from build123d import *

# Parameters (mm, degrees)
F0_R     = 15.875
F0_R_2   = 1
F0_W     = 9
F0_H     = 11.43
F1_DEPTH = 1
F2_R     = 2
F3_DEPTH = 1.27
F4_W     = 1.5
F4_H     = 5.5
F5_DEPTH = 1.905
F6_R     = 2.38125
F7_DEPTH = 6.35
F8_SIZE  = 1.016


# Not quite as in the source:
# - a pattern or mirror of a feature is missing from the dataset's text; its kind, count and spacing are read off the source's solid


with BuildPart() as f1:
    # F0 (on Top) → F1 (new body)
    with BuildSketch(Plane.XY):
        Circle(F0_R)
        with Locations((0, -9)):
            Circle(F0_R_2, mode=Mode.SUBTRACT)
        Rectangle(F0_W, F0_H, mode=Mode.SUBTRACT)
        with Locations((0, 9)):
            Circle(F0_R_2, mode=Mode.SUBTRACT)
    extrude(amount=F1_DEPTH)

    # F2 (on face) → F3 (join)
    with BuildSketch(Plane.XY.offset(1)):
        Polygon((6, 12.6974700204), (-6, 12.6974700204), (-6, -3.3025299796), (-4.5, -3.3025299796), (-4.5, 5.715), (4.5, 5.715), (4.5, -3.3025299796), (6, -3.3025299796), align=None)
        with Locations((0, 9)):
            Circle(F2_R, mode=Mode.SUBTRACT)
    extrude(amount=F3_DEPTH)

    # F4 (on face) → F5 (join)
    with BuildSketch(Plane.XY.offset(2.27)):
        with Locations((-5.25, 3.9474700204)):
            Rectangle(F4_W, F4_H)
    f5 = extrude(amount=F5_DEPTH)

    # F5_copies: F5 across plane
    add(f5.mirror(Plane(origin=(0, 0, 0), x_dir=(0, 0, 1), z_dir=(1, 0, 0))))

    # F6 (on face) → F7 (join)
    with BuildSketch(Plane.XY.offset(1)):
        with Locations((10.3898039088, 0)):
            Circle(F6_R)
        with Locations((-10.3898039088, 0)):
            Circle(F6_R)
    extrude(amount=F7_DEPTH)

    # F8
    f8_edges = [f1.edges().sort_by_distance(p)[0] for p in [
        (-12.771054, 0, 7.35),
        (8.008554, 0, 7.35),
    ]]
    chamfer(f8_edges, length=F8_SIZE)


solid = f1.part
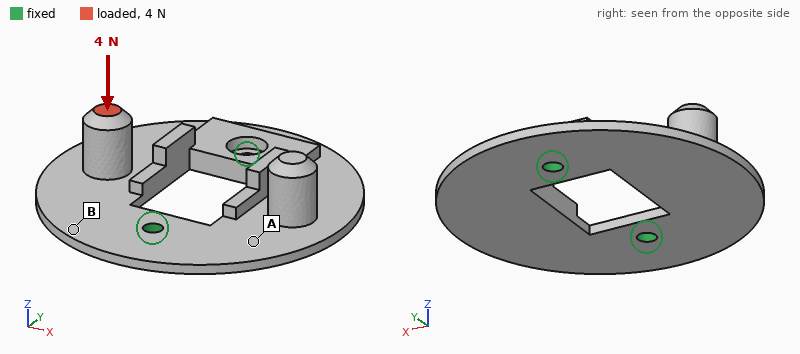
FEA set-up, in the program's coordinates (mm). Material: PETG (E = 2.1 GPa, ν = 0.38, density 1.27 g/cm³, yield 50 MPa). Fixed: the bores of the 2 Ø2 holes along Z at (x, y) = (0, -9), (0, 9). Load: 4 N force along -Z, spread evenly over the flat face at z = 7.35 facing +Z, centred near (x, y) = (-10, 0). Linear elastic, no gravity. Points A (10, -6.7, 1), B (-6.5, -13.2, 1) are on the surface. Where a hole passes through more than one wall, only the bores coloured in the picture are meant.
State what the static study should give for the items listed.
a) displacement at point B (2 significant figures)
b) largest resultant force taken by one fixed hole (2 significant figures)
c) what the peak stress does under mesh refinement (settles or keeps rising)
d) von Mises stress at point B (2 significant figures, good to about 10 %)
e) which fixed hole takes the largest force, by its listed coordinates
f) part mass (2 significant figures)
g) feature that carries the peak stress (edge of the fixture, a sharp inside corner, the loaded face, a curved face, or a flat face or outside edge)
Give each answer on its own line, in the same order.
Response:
0.087 mm
2.4 N
keeps rising
3.5 MPa
(0, 9)
1.3 g
edge of the fixture
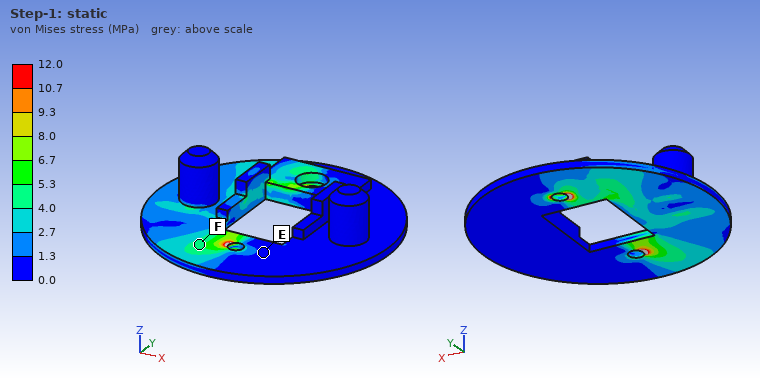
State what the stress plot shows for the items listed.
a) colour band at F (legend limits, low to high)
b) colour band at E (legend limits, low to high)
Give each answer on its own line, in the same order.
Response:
4.0 to 5.3 MPa
0.0 to 1.3 MPa
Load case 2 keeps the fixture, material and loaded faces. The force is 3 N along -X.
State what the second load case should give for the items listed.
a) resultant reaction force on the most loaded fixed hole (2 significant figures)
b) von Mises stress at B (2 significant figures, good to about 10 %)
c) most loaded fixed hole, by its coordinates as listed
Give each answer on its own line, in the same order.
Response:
1.8 N
2.8 MPa
(0, 9)
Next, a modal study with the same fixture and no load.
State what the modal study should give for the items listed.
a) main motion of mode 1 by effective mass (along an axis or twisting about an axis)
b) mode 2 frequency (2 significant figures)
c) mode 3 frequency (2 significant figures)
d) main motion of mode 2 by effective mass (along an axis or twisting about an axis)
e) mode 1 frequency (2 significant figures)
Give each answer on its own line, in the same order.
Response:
twisting about Y
980 Hz
2200 Hz
along Z
860 Hz
